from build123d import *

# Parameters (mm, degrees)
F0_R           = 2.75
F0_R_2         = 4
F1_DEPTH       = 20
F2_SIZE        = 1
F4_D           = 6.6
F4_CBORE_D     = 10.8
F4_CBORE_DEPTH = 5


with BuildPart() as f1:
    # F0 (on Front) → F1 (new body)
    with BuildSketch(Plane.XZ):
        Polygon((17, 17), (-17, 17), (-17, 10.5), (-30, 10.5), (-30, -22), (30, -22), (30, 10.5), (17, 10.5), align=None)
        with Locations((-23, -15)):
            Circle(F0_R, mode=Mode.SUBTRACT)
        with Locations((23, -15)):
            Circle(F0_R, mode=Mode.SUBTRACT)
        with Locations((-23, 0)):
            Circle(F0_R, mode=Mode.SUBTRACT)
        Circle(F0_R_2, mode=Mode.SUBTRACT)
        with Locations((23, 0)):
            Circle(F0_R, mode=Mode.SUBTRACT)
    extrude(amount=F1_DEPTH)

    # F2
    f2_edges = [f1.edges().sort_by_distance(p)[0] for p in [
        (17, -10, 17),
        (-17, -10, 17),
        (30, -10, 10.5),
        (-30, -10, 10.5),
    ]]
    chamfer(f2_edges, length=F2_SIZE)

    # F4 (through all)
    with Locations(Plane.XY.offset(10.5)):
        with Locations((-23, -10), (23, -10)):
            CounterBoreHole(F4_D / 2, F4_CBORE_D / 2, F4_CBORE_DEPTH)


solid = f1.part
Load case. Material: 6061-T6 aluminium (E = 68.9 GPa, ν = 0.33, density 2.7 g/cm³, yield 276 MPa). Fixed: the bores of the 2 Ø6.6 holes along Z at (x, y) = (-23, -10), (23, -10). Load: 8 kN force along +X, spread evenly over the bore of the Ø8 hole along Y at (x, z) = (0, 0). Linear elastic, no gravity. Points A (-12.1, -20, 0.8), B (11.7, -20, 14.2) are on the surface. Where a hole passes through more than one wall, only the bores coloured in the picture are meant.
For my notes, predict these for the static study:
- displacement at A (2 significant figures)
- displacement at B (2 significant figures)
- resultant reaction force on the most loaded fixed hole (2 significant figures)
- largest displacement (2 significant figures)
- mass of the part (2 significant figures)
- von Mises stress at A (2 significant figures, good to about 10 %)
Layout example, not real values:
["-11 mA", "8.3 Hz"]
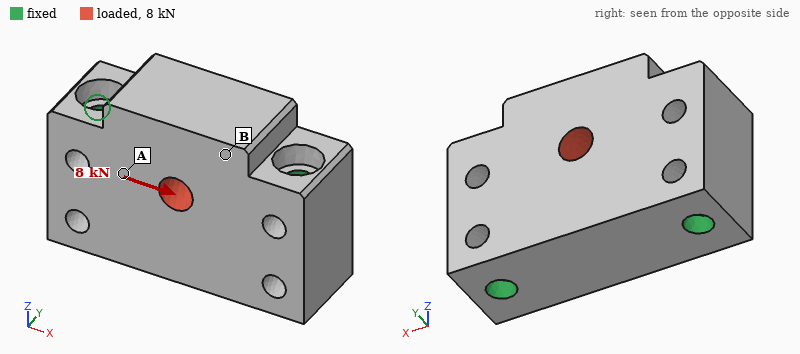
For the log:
["2.3 µm", "2.6 µm", "4.1 kN", "4.4 µm", "100 g", "11 MPa"]
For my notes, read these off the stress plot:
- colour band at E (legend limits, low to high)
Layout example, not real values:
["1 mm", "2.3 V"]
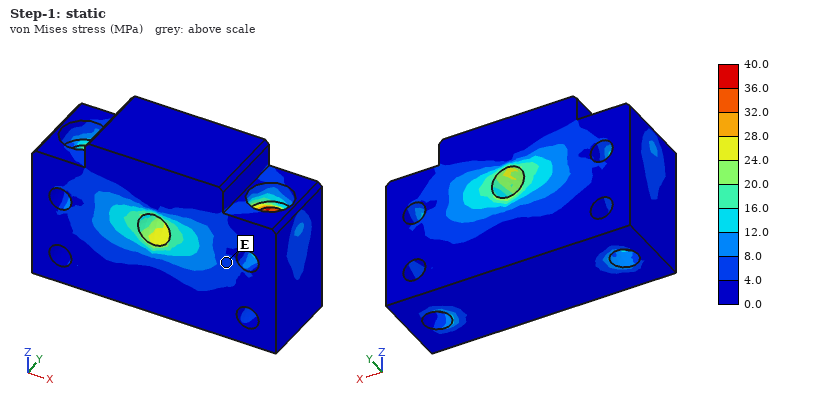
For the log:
["4.0 to 8.0 MPa"]
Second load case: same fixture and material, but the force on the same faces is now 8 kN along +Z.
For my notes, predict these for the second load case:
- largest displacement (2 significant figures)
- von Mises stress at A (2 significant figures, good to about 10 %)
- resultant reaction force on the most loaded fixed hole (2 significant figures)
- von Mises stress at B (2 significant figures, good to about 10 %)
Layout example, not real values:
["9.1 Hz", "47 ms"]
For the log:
["7.4 µm", "9.6 MPa", "4.1 kN", "7.1 MPa"]
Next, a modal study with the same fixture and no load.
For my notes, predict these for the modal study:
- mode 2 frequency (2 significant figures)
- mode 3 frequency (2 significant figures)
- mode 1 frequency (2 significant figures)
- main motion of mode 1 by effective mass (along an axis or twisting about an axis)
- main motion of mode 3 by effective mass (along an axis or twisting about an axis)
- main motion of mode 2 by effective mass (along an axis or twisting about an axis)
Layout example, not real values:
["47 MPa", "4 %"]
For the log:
["25 kHz", "27 kHz", "17 kHz", "along Y", "along Z", "along Y"]
